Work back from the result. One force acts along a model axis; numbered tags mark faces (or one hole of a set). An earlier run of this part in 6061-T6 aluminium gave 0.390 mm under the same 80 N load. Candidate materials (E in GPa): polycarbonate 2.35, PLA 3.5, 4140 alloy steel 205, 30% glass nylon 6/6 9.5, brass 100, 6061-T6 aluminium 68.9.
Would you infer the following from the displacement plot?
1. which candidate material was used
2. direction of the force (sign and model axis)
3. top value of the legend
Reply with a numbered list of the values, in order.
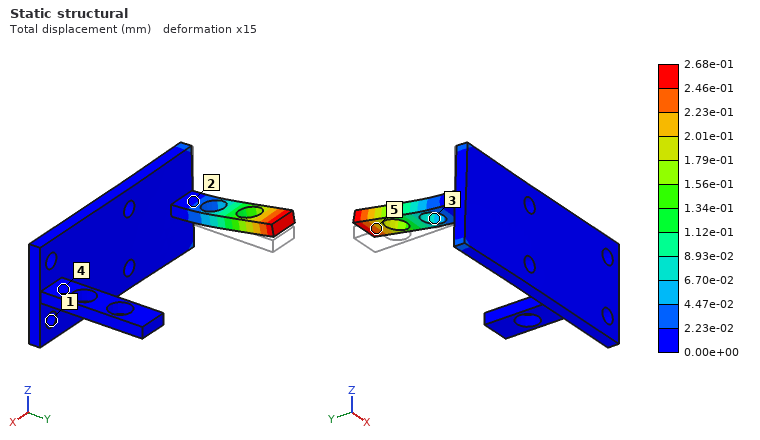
1. brass
2. +Z
3. 2.68e-01 mm
